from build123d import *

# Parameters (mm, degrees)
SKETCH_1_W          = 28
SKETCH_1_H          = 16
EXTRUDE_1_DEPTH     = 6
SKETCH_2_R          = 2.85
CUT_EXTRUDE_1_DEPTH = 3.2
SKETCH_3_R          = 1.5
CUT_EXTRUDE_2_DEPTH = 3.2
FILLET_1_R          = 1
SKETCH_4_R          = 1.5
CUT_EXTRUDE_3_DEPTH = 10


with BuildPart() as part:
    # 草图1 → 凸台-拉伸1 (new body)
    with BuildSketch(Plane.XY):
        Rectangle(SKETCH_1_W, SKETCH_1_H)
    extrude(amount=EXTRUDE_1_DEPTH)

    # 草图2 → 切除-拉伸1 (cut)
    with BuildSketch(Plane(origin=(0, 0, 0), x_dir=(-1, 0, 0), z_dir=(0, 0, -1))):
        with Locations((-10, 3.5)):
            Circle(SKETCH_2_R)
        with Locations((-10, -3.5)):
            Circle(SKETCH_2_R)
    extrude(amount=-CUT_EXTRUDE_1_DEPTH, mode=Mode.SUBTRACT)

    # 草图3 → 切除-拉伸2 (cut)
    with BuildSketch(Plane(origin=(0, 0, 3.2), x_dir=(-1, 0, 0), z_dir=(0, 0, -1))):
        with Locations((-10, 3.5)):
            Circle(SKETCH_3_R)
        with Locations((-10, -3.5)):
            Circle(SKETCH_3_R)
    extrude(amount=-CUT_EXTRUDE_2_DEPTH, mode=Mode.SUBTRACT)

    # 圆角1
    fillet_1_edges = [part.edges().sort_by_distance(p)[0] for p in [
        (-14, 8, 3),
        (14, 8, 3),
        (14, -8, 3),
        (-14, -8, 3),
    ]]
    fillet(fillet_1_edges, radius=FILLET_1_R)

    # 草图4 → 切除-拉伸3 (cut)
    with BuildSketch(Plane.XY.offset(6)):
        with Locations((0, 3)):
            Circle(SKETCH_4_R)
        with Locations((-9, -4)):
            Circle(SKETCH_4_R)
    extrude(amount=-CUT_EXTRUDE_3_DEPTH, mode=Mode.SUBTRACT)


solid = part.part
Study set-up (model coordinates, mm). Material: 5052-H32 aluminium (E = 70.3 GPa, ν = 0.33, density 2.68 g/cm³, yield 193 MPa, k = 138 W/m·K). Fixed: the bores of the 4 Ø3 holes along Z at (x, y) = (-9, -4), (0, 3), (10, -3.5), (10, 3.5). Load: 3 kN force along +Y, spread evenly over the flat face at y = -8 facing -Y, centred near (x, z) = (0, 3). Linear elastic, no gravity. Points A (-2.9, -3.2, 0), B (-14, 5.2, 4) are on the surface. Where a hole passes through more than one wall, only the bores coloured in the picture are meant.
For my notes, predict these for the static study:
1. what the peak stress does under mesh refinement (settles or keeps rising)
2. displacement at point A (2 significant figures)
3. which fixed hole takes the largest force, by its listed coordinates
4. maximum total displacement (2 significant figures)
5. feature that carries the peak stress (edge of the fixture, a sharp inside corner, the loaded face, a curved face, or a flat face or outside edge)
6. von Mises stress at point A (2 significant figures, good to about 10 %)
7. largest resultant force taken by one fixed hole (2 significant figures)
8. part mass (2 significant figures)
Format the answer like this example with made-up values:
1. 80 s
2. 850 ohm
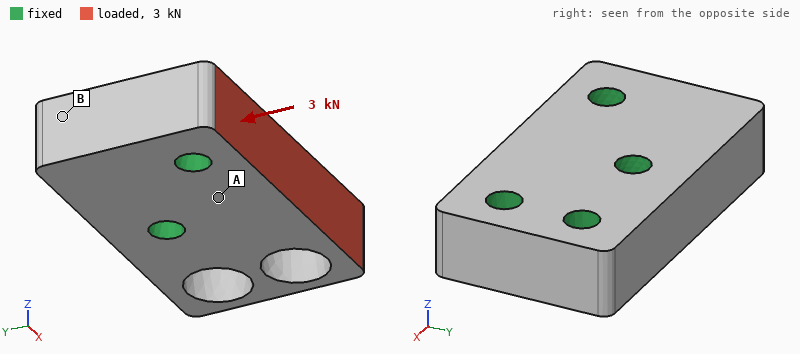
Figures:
1. keeps rising
2. 1.7 µm
3. (-9, -4)
4. 7.7 µm
5. edge of the fixture
6. 16 MPa
7. 1.1 kN
8. 6.4 g
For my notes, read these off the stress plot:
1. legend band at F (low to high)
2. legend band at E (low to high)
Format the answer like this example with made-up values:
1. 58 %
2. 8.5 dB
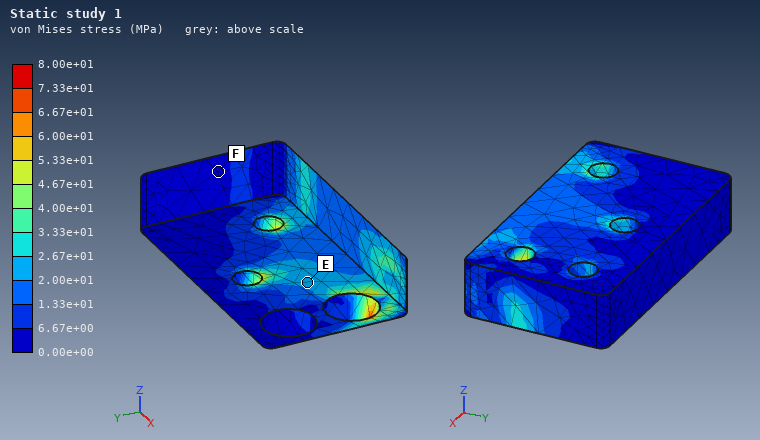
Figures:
1. 0.00e+00 to 6.67e+00 MPa
2. 2.00e+01 to 2.67e+01 MPa
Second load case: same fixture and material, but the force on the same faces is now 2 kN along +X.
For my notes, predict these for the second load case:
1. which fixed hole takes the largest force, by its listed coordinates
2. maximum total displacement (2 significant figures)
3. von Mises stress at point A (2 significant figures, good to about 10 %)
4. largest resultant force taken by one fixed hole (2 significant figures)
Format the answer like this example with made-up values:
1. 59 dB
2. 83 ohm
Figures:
1. (-9, -4)
2. 5.6 µm
3. 12 MPa
4. 1.2 kN
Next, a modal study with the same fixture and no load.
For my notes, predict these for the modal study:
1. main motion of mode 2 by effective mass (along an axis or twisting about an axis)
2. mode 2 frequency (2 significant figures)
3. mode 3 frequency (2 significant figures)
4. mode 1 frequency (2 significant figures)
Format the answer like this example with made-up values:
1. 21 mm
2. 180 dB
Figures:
1. along Z
2. 63 kHz
3. 83 kHz
4. 45 kHz
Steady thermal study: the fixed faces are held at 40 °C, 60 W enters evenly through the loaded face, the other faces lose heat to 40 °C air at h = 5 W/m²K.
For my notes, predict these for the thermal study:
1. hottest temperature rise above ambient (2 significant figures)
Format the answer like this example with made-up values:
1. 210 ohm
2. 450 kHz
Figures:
1. 22 K
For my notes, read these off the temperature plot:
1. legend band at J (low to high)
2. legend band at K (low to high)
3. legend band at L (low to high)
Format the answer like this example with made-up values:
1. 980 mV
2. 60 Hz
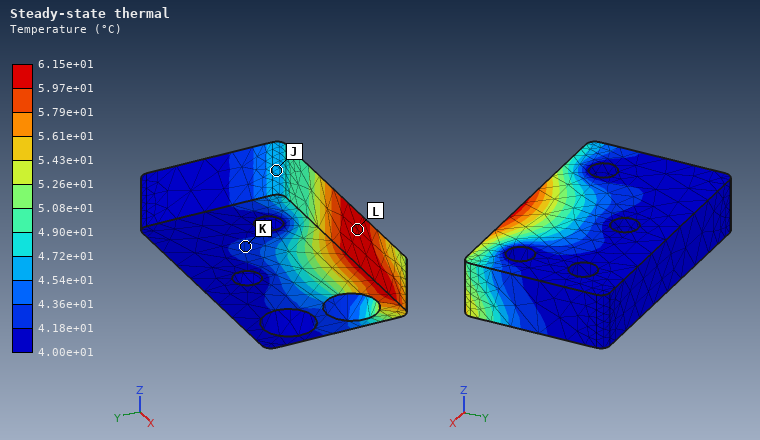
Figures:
1. 4.54e+01 to 4.72e+01 °C
2. 4.18e+01 to 4.36e+01 °C
3. 5.97e+01 to 6.15e+01 °C
